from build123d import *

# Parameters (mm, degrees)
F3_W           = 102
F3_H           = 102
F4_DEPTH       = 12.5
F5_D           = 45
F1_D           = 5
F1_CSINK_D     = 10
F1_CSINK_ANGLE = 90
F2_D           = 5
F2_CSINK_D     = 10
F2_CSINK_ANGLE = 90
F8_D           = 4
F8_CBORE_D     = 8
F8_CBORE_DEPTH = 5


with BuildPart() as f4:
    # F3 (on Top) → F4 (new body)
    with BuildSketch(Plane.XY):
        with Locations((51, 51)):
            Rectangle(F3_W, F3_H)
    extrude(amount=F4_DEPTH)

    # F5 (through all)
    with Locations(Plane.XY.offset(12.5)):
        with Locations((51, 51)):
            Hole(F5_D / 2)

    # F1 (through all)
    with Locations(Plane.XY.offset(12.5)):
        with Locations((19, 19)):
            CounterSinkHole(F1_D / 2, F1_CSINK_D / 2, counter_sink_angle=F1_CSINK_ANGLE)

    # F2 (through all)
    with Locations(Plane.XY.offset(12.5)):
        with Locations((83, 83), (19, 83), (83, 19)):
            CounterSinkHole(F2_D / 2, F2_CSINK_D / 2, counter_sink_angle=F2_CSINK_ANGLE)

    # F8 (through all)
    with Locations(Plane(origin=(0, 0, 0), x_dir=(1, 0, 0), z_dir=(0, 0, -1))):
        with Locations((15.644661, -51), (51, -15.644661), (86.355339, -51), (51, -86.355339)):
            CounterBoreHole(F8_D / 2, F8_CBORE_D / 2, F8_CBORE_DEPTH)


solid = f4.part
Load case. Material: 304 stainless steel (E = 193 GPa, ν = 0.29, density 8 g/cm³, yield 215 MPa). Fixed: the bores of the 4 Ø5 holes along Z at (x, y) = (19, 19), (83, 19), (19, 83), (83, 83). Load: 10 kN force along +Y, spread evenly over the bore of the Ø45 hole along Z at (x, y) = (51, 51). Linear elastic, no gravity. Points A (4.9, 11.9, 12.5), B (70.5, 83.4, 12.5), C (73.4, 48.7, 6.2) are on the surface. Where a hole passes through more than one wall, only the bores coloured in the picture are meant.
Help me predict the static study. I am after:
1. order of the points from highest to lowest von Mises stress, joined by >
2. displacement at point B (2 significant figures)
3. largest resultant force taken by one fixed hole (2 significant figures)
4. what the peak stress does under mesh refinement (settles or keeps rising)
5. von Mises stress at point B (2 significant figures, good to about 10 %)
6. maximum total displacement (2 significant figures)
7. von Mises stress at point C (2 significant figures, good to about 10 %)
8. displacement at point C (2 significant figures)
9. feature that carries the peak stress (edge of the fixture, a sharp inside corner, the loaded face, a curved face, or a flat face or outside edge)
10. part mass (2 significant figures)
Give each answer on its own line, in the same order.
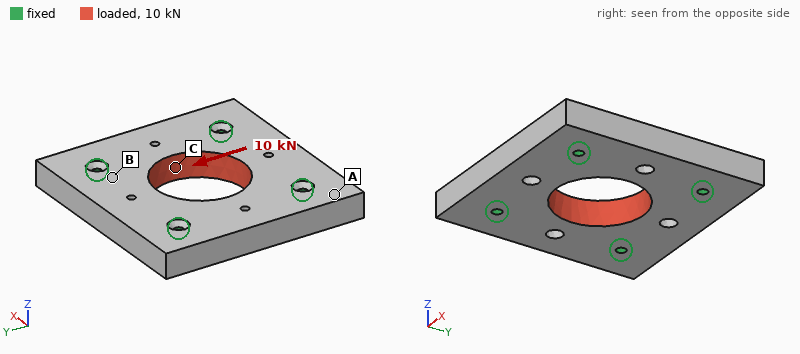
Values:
C > B > A
1.2 µm
2.5 kN
keeps rising
6.1 MPa
2.3 µm
10.0 MPa
1.2 µm
edge of the fixture
860 g
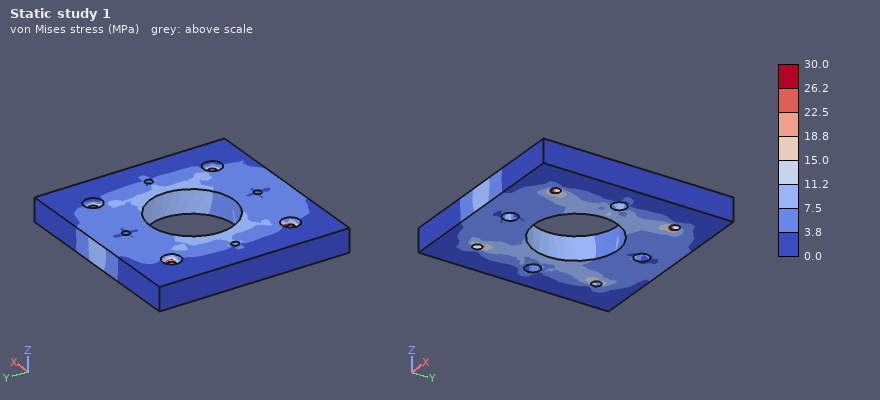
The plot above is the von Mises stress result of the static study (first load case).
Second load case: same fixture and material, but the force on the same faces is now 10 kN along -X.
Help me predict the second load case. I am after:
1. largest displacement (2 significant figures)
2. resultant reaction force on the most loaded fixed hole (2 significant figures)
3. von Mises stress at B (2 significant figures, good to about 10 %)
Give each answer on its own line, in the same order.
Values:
2.3 µm
2.5 kN
6.0 MPa
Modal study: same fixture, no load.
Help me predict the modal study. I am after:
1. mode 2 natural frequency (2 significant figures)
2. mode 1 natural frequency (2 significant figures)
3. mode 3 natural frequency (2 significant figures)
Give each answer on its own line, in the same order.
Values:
9900 Hz
8500 Hz
9900 Hz
